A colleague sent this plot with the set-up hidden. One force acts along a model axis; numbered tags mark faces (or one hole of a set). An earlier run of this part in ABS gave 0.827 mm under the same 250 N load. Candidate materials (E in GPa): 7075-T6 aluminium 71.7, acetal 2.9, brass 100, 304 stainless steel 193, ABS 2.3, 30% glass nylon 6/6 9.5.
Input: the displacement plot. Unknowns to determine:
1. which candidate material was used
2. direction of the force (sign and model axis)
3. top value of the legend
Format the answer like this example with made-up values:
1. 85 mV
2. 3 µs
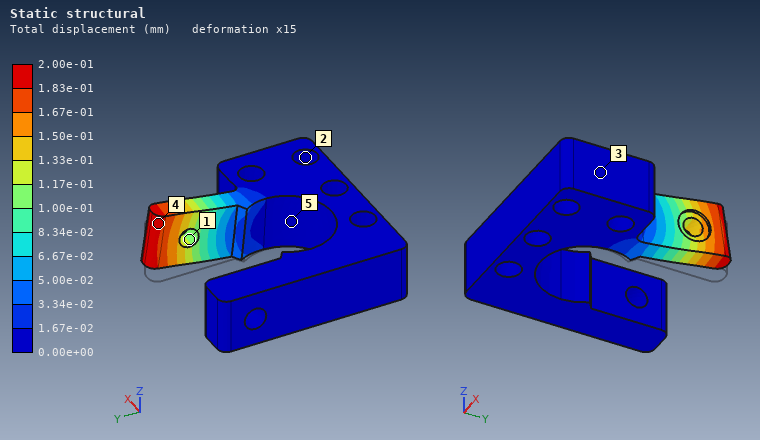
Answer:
1. 30% glass nylon 6/6
2. +Z
3. 2.00e-01 mm
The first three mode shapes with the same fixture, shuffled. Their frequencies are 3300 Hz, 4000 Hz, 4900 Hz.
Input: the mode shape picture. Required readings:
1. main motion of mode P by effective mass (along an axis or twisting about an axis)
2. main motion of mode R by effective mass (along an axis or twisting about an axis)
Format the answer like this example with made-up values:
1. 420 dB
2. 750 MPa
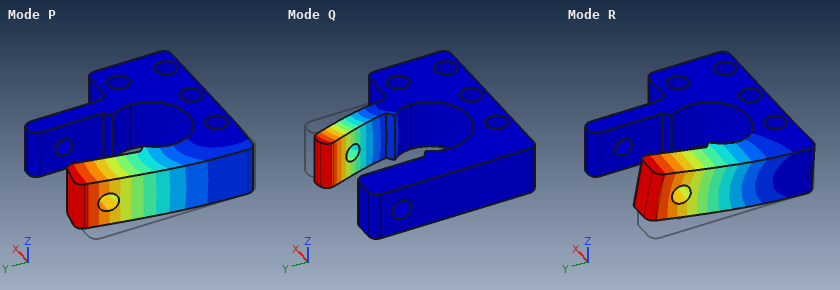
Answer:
1. along X
2. along Z
